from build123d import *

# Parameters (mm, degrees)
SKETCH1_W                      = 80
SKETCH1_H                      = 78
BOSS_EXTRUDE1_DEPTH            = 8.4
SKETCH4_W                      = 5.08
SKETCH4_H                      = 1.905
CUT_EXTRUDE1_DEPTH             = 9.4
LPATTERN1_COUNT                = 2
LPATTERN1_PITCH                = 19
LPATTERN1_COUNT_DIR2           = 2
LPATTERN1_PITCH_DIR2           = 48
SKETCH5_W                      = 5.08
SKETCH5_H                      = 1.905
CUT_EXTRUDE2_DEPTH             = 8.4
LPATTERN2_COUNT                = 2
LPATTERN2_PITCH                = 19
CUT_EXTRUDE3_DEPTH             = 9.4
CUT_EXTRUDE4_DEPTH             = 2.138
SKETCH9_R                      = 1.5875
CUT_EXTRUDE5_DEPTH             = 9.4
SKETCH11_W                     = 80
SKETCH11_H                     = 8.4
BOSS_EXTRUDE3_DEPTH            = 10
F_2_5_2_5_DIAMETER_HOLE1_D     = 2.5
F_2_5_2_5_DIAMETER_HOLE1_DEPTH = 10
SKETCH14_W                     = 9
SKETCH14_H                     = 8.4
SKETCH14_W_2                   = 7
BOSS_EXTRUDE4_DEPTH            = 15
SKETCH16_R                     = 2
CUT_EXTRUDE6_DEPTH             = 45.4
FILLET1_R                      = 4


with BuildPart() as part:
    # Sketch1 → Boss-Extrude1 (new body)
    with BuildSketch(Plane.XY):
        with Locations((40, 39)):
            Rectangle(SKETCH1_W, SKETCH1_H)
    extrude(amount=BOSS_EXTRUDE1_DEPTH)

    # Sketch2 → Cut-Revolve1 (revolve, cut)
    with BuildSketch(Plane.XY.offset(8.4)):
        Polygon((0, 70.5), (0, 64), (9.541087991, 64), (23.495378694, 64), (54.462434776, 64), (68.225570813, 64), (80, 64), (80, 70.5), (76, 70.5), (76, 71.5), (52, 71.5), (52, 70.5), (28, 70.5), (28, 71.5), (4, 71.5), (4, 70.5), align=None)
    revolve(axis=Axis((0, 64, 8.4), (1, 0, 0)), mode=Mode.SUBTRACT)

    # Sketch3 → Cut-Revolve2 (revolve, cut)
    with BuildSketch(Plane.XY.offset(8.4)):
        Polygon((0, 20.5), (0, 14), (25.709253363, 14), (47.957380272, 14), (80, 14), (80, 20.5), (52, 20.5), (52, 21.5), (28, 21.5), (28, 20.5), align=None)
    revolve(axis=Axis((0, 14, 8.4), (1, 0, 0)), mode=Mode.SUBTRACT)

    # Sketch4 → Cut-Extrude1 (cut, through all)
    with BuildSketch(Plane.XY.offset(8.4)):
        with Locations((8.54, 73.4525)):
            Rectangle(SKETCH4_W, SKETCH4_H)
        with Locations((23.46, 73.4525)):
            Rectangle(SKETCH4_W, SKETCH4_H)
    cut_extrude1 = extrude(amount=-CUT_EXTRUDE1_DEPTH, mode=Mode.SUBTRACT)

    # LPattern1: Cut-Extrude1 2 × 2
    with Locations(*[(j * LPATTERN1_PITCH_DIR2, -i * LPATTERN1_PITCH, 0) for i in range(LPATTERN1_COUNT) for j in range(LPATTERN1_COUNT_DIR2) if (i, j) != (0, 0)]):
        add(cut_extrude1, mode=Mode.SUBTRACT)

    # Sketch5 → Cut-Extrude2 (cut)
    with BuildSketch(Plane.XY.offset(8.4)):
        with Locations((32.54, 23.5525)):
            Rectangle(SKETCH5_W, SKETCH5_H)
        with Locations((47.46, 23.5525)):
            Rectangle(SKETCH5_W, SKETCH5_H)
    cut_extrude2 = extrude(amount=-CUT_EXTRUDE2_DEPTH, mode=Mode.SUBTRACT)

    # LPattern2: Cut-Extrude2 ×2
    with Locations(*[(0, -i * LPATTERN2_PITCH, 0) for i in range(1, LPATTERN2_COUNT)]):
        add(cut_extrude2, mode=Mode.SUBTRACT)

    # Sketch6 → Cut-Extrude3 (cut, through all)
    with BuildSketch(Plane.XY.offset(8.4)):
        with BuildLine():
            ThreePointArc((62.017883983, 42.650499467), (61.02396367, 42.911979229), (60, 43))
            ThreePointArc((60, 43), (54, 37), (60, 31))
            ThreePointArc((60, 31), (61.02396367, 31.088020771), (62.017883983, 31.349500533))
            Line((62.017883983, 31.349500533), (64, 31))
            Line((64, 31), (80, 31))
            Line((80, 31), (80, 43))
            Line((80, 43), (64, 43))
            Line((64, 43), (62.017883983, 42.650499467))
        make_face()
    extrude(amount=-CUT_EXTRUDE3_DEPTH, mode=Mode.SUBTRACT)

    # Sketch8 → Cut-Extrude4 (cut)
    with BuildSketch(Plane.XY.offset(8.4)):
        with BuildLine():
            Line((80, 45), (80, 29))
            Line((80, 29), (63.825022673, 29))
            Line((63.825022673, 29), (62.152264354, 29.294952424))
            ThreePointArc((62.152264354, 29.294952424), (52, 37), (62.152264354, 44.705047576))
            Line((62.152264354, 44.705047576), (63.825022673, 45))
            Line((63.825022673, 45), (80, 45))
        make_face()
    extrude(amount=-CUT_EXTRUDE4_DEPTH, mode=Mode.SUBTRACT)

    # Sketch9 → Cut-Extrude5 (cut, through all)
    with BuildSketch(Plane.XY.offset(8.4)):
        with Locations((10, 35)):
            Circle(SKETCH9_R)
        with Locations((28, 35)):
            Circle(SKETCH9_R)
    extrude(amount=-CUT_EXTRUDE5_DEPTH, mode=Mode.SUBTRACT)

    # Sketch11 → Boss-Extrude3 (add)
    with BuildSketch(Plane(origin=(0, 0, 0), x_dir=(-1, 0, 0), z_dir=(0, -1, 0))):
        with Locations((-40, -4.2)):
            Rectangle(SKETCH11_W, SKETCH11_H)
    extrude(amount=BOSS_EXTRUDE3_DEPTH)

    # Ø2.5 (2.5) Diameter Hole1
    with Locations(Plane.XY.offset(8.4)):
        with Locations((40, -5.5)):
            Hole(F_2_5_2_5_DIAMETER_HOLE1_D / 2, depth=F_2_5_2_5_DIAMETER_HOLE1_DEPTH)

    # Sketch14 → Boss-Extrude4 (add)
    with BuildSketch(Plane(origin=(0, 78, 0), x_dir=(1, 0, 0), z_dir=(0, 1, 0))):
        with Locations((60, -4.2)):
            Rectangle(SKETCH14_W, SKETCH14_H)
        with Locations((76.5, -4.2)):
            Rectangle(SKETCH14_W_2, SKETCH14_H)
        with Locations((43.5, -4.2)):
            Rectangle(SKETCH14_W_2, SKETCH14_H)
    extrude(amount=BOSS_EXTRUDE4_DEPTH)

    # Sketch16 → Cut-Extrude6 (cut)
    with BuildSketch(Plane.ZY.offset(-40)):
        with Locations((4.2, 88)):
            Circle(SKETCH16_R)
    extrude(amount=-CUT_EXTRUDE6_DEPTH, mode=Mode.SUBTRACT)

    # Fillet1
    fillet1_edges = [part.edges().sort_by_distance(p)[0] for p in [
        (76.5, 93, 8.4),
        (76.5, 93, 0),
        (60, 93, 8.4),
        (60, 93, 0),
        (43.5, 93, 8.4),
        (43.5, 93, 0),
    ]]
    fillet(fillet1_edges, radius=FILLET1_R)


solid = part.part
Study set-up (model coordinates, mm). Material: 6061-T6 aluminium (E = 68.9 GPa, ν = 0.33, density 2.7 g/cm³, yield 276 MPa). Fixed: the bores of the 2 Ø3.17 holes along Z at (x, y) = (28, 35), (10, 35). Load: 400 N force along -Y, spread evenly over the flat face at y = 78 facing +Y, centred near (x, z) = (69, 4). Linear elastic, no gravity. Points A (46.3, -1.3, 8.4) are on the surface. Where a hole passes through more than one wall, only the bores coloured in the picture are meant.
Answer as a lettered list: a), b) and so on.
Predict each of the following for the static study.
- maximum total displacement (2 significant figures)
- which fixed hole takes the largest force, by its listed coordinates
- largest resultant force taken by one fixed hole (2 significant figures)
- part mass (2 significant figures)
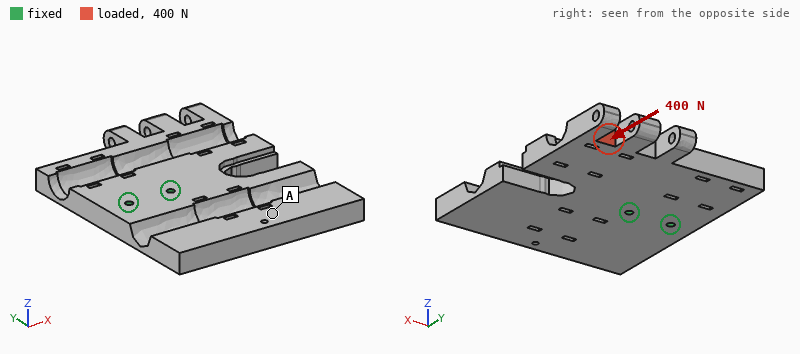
a) 0.14 mm
b) (28, 35)
c) 1.2 kN
d) 120 g
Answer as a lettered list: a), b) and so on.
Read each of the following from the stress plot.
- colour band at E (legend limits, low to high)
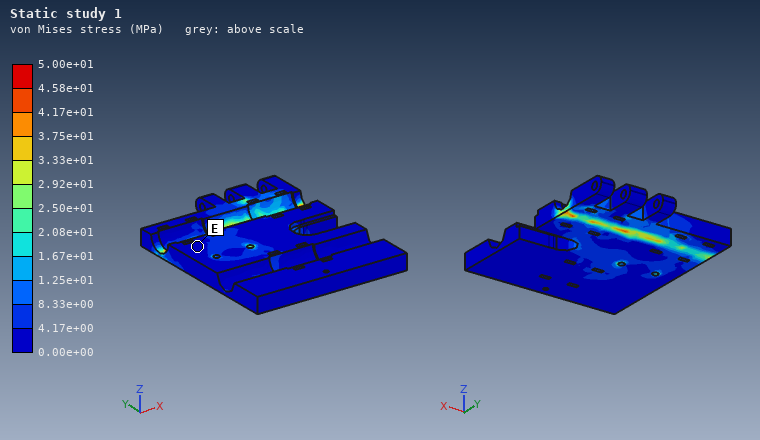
a) 0.00e+00 to 4.17e+00 MPa
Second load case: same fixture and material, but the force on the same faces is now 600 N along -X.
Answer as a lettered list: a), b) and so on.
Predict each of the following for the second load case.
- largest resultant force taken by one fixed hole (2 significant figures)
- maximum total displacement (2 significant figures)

a) 1.3 kN
b) 48 µm
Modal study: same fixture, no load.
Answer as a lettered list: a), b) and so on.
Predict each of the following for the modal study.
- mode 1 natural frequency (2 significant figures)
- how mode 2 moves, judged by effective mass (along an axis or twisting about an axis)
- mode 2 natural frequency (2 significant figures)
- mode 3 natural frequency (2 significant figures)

a) 990 Hz
b) along Z
c) 1100 Hz
d) 2100 Hz
